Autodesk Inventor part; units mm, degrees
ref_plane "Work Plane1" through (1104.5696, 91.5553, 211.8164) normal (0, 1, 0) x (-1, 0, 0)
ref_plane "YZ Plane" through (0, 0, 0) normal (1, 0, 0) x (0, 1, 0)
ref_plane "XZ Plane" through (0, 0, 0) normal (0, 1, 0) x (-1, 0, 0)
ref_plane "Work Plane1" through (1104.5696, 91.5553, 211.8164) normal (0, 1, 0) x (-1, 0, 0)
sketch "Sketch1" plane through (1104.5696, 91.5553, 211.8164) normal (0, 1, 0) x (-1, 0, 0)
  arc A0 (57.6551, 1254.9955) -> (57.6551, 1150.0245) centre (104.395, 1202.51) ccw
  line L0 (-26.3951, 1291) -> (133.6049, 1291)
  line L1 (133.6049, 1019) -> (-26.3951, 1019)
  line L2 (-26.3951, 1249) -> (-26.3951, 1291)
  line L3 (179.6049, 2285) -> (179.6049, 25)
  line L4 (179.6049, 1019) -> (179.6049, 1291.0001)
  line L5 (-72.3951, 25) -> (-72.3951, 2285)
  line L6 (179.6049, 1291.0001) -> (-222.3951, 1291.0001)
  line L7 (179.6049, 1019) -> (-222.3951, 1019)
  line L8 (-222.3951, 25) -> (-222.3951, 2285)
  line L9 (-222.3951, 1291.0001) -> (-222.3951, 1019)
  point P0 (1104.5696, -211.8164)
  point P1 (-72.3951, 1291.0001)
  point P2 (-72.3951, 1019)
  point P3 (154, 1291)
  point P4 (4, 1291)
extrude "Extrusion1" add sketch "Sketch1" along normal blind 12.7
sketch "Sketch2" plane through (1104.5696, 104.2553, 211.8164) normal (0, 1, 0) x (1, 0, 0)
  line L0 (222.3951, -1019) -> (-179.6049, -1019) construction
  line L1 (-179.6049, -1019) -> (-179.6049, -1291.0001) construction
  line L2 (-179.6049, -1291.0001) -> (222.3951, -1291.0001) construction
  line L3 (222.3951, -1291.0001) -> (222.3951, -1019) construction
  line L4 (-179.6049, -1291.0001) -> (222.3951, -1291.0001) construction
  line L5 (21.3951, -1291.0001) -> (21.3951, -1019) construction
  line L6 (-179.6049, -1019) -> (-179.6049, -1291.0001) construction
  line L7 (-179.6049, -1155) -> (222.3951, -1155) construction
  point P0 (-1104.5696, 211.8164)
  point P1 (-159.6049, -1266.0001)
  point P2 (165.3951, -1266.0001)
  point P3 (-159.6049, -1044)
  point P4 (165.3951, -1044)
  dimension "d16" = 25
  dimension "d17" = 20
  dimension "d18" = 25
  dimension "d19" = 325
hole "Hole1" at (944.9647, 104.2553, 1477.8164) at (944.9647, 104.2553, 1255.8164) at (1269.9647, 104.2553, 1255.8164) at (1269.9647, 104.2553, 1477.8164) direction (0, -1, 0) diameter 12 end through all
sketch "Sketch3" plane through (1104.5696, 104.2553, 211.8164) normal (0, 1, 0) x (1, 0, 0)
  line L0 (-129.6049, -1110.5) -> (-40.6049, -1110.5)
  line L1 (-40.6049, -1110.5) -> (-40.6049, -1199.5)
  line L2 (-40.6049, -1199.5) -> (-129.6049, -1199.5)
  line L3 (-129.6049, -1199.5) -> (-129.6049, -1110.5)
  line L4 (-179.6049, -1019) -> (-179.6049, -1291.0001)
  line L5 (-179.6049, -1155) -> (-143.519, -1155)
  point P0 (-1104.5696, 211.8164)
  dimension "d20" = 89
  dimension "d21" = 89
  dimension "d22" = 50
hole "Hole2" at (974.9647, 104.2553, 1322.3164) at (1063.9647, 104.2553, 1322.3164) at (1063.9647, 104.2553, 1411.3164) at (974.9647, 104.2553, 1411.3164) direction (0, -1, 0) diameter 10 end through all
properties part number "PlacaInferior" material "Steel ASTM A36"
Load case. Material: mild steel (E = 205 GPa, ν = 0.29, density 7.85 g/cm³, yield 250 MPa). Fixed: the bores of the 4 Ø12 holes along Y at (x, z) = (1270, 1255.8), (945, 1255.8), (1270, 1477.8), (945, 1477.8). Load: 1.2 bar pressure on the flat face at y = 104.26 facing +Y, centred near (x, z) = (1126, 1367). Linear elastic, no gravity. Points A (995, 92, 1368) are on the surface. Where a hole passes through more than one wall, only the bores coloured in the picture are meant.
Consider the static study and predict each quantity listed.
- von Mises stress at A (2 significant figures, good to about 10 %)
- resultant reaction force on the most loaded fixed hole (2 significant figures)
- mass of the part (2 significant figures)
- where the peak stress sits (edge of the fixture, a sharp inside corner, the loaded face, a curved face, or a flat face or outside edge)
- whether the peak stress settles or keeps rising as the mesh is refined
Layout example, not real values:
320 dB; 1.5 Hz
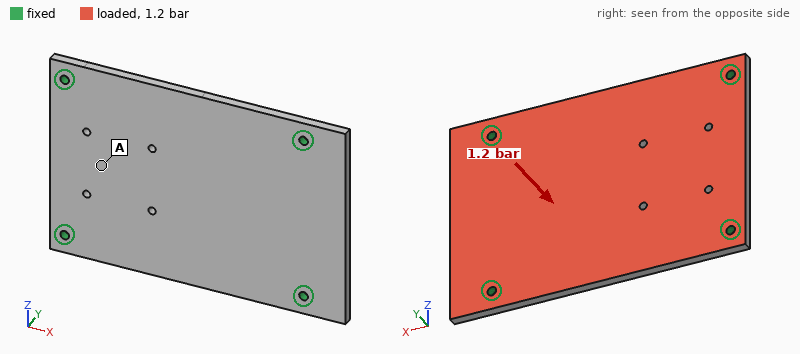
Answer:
13 MPa; 3.6 kN; 11 kg; edge of the fixture; keeps rising
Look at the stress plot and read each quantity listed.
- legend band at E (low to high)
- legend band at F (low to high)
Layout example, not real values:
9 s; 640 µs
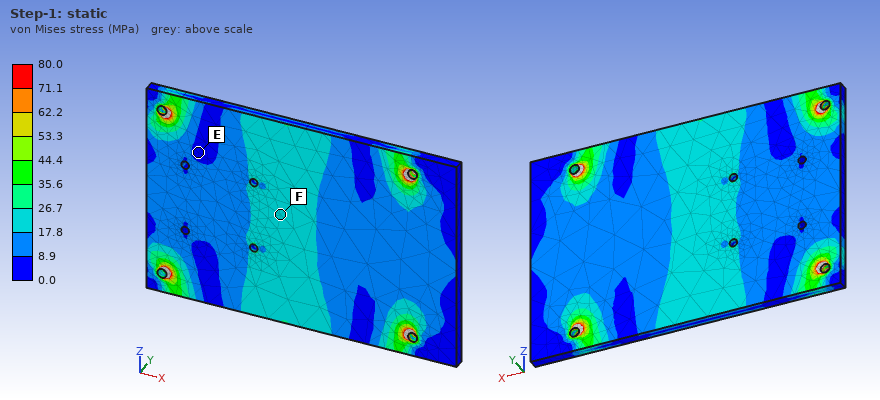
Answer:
0.0 to 8.9 MPa; 17.8 to 26.7 MPa
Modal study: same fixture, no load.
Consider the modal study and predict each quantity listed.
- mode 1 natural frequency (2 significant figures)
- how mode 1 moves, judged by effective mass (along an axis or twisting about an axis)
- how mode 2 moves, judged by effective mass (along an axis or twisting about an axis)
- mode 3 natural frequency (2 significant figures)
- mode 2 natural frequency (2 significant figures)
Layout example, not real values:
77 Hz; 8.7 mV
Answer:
500 Hz; along Y; twisting about X; 1100 Hz; 780 Hz
